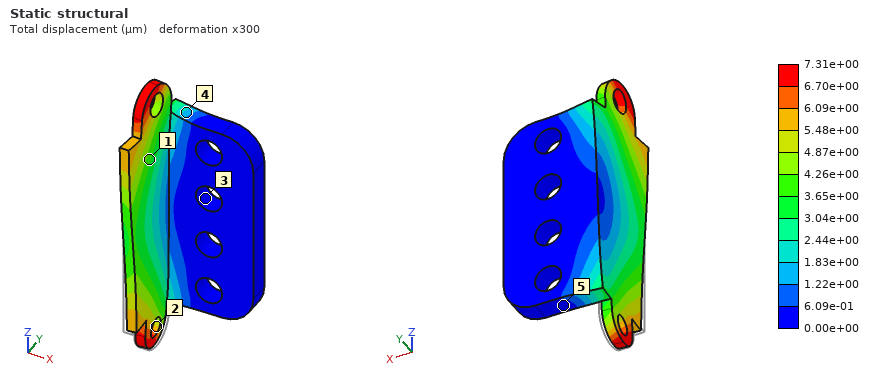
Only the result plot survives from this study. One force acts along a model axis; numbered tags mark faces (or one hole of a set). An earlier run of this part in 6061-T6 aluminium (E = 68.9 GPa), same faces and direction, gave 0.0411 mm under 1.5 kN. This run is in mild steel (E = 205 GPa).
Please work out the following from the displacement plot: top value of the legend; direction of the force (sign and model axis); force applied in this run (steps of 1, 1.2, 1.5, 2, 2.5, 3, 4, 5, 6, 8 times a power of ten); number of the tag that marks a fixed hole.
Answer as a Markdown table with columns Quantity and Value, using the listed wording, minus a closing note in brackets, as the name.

| Quantity | Value |
|---|---|
| top value of the legend | 7.31e+00 µm |
| direction of the force | +Z |
| force applied in this run | 800 N |
| number of the tag that marks a fixed hole | 3 |
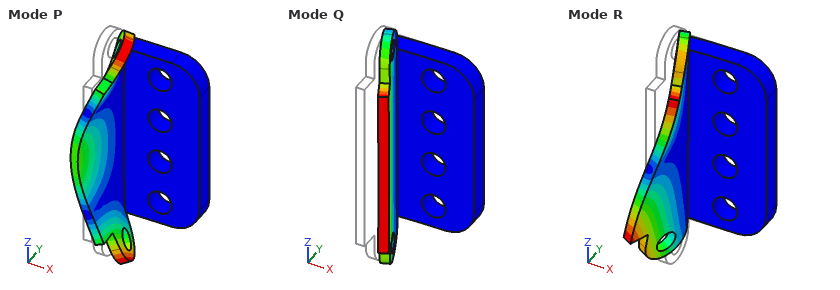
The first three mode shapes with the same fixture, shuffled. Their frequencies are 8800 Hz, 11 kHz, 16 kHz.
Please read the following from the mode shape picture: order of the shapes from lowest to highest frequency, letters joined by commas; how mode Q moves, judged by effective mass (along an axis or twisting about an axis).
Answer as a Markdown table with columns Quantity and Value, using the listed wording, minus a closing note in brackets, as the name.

| Quantity | Value |
|---|---|
| order of the shapes from lowest to highest frequency, letters joined by commas | Q, R, P |
| how mode Q moves, judged by effective mass | along X |
